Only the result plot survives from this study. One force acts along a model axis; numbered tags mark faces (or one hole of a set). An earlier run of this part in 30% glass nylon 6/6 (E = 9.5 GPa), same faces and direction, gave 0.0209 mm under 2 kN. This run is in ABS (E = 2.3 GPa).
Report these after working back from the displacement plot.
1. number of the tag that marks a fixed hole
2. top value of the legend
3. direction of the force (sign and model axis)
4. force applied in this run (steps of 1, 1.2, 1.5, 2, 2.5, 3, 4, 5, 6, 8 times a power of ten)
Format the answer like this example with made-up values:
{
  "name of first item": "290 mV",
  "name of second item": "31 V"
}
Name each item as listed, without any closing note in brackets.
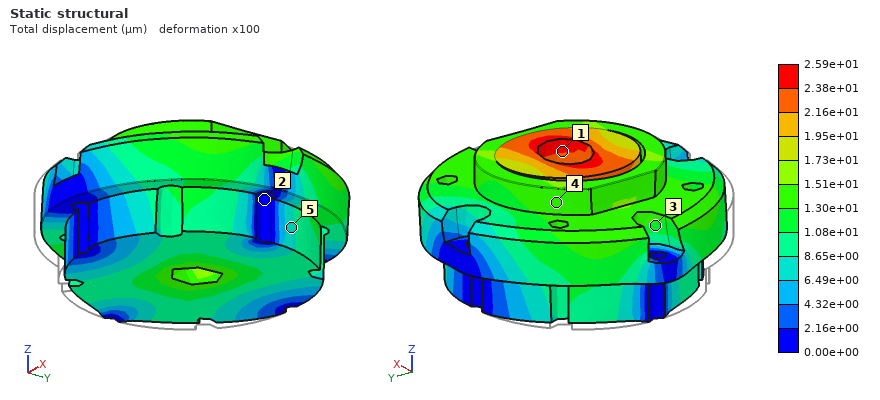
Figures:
{
  "number of the tag that marks a fixed hole": "2",
  "top value of the legend": "2.59e+01 µm",
  "direction of the force": "+X",
  "force applied in this run": "600 N"
}
